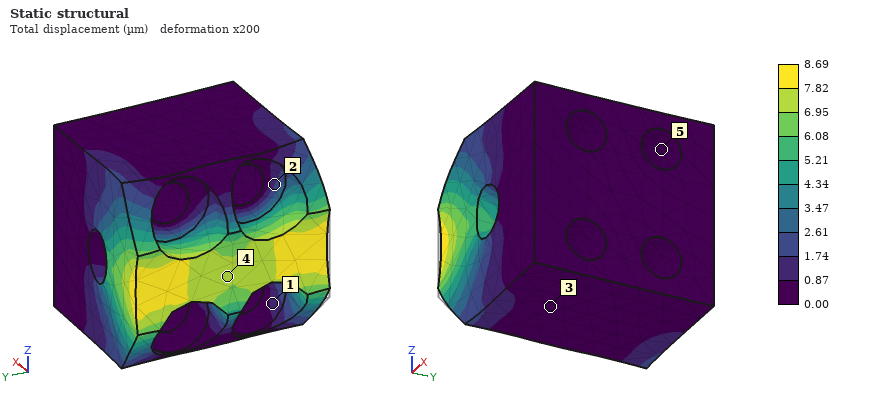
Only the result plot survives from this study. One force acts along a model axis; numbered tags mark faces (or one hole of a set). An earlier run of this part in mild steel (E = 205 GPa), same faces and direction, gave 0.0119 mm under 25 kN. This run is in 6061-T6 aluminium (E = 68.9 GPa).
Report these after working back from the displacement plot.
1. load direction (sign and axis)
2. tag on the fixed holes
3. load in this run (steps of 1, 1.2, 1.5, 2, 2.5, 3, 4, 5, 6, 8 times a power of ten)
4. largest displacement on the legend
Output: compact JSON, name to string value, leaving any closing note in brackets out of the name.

{"load direction": "+X", "tag on the fixed holes": "5", "load in this run": "6 kN", "largest displacement on the legend": "8.69 µm"}
